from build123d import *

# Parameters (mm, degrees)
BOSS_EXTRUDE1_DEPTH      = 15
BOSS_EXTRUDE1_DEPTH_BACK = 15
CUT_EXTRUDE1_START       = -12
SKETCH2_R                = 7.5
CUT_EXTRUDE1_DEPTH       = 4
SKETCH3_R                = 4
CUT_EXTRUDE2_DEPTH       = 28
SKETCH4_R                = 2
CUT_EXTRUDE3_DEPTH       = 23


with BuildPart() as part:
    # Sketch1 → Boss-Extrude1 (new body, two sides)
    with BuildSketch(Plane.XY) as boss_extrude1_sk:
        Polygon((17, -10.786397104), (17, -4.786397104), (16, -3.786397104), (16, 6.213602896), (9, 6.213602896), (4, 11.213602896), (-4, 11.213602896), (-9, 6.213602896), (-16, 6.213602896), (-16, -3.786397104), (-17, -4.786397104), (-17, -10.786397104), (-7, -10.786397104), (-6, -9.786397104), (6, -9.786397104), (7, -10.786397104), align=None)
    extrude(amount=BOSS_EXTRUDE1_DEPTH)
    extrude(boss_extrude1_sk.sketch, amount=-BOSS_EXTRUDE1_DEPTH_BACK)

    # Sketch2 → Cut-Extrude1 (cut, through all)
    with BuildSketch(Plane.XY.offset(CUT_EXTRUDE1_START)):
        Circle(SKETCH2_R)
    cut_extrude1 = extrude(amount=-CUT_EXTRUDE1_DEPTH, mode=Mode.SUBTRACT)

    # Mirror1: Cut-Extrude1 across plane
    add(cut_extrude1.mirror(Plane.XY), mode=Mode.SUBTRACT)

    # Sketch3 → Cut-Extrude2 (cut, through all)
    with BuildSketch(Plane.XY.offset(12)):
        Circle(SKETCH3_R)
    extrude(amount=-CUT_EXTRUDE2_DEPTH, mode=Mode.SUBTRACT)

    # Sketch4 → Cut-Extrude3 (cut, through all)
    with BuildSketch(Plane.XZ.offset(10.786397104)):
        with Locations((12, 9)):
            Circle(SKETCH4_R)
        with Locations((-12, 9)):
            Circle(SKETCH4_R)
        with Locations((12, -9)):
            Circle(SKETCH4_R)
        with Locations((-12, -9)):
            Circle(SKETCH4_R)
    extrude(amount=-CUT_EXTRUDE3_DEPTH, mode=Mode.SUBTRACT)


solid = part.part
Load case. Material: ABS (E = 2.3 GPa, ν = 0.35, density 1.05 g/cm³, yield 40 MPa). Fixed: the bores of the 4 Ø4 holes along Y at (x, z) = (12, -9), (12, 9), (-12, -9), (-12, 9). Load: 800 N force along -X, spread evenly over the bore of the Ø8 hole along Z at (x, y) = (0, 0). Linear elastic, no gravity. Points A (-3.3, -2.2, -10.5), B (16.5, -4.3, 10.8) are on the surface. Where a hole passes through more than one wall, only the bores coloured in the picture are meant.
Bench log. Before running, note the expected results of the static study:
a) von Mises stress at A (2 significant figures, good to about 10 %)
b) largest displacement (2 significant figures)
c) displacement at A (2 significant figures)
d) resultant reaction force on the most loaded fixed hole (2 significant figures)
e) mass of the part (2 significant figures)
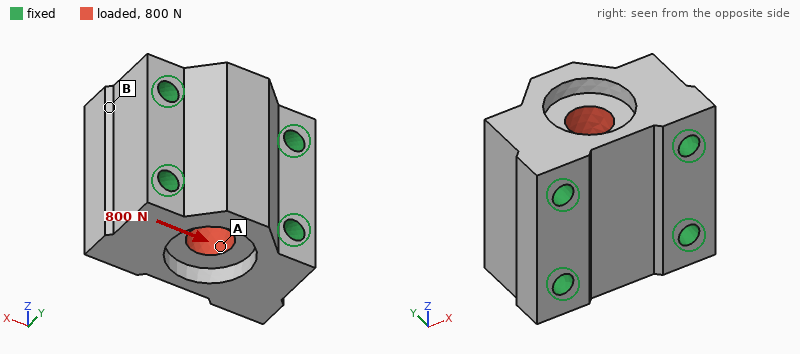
1.6 MPa
8.0 µm
4.0 µm
210 N
16 g
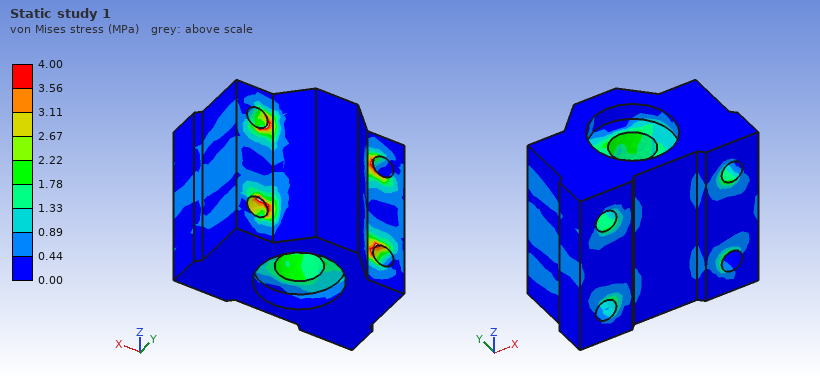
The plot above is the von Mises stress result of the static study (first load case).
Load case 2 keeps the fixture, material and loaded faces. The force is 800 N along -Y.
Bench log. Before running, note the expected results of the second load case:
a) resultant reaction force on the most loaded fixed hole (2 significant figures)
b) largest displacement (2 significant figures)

200 N
15 µm
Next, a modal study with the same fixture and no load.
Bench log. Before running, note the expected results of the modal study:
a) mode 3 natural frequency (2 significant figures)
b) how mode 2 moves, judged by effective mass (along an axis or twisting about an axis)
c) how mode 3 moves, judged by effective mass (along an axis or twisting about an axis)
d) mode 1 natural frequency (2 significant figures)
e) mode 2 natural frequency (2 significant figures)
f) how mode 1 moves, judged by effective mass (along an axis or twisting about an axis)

20 kHz
along Y
along Z
15 kHz
17 kHz
along Z
